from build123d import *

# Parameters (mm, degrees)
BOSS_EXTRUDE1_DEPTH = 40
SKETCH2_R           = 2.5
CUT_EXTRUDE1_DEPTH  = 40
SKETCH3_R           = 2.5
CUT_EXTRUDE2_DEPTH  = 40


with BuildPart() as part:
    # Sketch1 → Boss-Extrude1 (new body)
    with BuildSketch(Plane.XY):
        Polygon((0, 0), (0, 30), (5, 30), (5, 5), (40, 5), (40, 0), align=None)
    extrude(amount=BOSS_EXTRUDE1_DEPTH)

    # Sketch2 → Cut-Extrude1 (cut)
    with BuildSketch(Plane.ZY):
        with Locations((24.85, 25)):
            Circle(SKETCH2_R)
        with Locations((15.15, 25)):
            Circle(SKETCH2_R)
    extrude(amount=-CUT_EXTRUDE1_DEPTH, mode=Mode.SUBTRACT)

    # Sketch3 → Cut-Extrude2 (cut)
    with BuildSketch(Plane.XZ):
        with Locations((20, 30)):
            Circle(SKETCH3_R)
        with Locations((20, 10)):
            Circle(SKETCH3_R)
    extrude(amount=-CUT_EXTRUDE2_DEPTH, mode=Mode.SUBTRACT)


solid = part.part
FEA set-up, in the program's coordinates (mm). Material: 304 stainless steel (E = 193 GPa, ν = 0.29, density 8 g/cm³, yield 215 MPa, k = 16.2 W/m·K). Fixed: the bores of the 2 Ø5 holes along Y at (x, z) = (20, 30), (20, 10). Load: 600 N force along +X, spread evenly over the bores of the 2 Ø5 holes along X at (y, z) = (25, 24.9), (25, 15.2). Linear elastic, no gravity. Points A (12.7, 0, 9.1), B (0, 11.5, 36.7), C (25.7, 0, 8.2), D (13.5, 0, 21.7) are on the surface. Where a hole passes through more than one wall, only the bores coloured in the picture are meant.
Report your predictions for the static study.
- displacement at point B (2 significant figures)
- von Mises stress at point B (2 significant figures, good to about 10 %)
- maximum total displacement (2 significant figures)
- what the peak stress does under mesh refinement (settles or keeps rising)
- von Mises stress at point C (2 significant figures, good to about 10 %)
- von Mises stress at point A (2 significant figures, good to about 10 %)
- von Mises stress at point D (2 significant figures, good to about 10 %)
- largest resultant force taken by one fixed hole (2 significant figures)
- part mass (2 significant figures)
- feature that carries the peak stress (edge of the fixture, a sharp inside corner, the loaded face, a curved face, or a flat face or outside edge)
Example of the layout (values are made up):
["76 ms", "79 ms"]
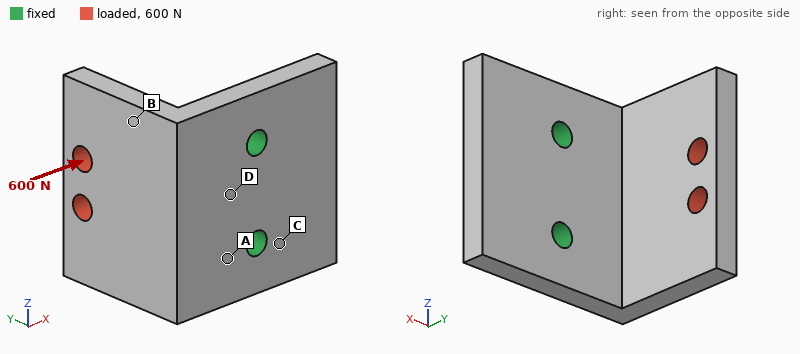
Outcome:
["0.042 mm", "49 MPa", "0.11 mm", "keeps rising", "9.0 MPa", "75 MPa", "64 MPa", "320 N", "100 g", "edge of the fixture"]
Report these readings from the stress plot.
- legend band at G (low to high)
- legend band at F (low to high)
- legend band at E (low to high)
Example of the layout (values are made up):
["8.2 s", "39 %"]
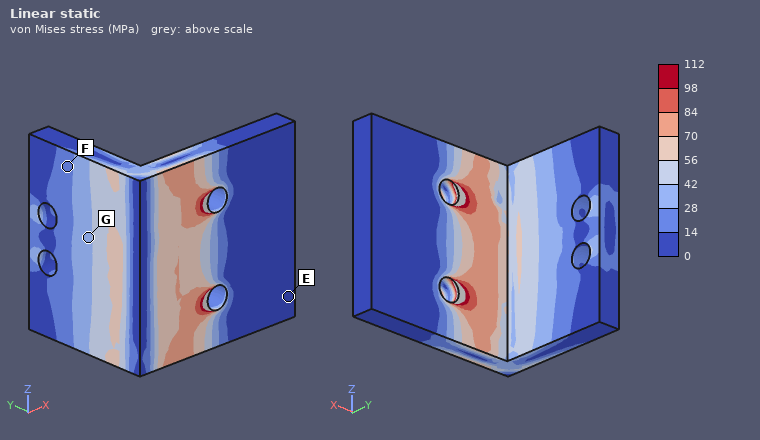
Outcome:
["28 to 42 MPa", "14 to 28 MPa", "0 to 14 MPa"]
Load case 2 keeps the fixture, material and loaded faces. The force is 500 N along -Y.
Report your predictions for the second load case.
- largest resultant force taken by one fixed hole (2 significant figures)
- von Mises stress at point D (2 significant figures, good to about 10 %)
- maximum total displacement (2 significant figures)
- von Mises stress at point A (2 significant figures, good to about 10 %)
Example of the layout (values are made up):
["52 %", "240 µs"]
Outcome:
["250 N", "26 MPa", "28 µm", "31 MPa"]
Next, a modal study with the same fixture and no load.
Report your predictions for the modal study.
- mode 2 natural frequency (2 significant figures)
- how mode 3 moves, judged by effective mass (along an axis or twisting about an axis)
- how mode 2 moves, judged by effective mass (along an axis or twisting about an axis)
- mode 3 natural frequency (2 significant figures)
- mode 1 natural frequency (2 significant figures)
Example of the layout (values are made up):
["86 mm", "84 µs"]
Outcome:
["4800 Hz", "along Y", "along Z", "7800 Hz", "2700 Hz"]
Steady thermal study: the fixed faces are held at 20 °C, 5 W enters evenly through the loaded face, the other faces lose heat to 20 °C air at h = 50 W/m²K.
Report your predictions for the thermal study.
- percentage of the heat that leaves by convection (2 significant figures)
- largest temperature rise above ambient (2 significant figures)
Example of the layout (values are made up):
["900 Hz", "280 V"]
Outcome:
["64 %", "41 K"]
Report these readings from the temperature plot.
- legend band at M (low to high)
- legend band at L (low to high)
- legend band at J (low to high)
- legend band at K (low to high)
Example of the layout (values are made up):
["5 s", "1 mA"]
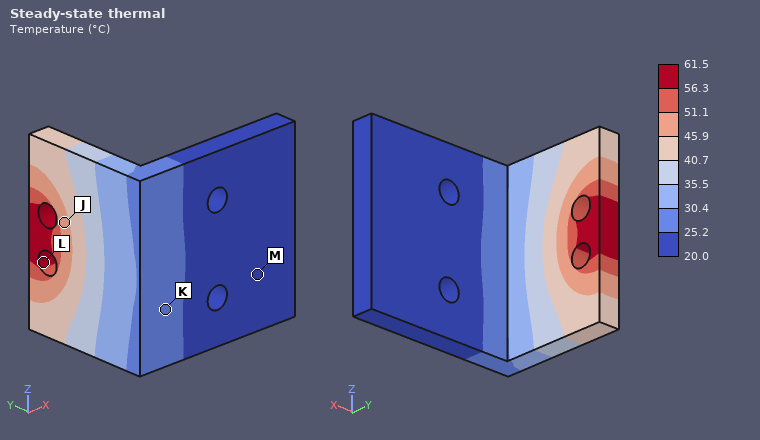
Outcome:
["20.0 to 25.2 °C", "56.3 to 61.5 °C", "45.9 to 51.1 °C", "25.2 to 30.4 °C"]
